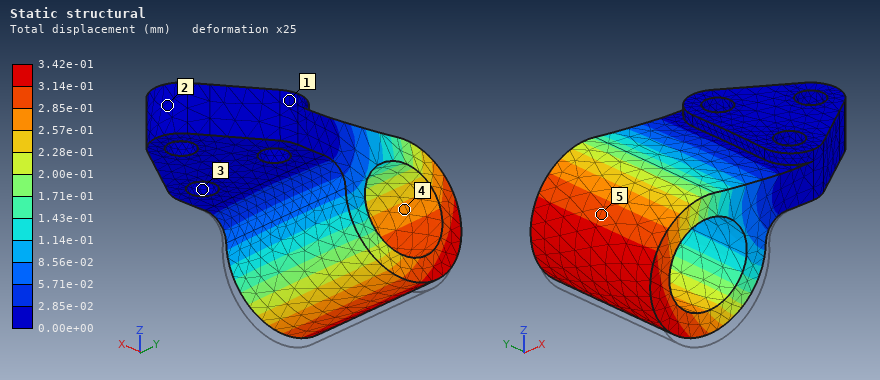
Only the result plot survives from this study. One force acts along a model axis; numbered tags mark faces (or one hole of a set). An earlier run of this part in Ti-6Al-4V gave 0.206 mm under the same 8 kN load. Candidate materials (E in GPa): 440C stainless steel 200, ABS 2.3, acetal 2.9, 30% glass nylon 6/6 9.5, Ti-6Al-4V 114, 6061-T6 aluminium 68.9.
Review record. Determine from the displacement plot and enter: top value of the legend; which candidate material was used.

3.42e-01 mm
6061-T6 aluminium
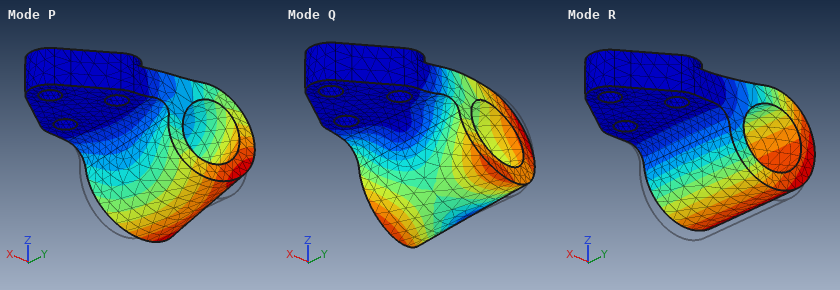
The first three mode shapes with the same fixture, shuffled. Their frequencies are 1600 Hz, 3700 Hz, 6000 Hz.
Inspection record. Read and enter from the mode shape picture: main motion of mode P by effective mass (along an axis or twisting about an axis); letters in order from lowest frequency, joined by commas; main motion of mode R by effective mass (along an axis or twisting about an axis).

along Y
R, P, Q
along Z
